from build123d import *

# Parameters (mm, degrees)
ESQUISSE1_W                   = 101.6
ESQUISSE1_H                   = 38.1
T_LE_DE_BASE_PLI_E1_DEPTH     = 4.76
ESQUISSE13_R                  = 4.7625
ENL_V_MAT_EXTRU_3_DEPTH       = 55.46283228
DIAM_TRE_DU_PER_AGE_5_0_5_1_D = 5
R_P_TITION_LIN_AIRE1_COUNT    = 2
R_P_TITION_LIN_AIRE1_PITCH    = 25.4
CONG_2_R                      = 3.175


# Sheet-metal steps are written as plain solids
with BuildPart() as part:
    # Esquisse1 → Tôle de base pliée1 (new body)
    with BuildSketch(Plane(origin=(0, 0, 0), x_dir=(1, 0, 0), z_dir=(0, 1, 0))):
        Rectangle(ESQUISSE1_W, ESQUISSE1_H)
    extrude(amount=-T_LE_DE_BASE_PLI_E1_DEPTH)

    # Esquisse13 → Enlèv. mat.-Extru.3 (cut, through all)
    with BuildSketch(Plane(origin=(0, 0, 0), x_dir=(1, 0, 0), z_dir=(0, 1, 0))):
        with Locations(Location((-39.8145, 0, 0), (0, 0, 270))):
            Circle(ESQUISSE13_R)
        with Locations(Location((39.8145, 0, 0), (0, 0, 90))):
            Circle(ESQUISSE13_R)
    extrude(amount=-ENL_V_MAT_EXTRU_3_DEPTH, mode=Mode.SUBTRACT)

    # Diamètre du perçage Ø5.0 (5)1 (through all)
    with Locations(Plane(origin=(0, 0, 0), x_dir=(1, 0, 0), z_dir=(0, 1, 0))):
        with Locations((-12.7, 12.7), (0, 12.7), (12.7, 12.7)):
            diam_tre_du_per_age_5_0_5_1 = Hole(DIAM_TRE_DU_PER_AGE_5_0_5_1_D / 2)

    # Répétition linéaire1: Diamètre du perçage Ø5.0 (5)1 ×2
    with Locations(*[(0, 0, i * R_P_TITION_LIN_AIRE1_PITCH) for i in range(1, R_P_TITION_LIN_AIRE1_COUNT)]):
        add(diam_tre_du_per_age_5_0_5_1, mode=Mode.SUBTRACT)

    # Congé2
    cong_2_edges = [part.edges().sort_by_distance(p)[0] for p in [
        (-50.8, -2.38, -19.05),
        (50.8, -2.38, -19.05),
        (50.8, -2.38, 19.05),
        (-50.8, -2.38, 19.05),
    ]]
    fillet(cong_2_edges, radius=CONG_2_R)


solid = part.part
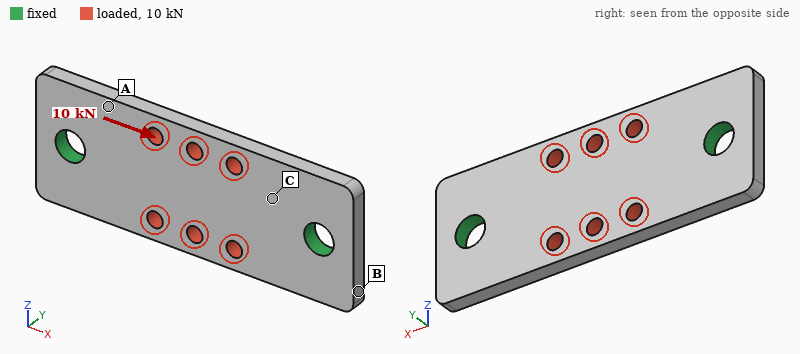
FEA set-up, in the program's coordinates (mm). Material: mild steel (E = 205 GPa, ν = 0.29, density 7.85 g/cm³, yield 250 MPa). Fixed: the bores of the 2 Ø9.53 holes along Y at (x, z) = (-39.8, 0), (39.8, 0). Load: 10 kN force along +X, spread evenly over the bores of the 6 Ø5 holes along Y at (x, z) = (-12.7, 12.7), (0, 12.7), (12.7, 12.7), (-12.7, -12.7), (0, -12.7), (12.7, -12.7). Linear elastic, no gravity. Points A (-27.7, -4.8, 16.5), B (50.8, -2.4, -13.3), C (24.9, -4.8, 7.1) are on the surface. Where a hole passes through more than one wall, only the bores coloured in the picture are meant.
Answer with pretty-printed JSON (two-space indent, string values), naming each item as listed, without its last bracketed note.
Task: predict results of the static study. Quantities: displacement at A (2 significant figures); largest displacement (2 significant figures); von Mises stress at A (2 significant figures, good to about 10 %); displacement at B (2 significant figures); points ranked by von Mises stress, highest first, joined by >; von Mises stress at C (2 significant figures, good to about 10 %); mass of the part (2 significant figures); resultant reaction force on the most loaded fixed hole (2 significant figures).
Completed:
{
  "displacement at A": "3.3 µm",
  "largest displacement": "6.3 µm",
  "von Mises stress at A": "19 MPa",
  "displacement at B": "2.2 µm",
  "points ranked by von Mises stress, highest first, joined by >": "C > A > B",
  "von Mises stress at C": "33 MPa",
  "mass of the part": "130 g",
  "resultant reaction force on the most loaded fixed hole": "5.0 kN"
}
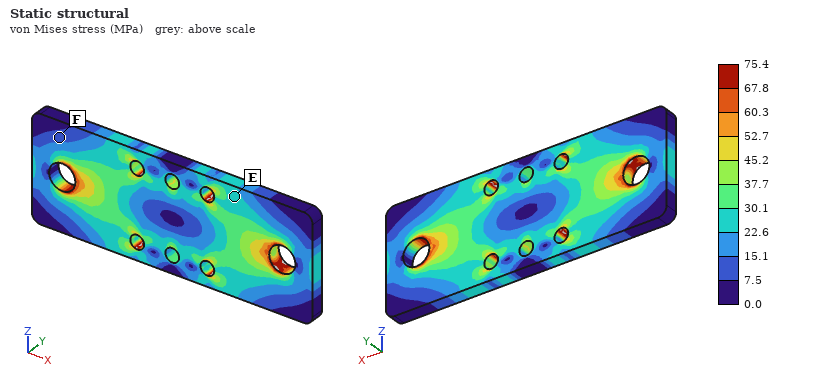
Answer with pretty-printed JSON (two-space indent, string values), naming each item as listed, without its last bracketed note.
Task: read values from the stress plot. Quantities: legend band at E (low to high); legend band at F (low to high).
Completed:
{
  "legend band at E": "22.6 to 30.1 MPa",
  "legend band at F": "7.5 to 15.1 MPa"
}
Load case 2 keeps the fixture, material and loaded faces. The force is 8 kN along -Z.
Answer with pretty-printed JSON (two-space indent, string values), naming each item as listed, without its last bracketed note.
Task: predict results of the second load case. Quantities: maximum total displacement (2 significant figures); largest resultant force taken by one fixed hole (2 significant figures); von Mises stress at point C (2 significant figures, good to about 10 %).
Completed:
{
  "maximum total displacement": "21 µm",
  "largest resultant force taken by one fixed hole": "4.0 kN",
  "von Mises stress at point C": "47 MPa"
}
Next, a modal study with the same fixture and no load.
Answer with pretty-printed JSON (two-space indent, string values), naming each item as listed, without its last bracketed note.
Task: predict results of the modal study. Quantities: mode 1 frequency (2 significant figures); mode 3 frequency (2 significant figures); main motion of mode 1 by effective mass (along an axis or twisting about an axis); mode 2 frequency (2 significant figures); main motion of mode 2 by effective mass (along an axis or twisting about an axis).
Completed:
{
  "mode 1 frequency": "4200 Hz",
  "mode 3 frequency": "10 kHz",
  "main motion of mode 1 by effective mass": "along Y",
  "mode 2 frequency": "5500 Hz",
  "main motion of mode 2 by effective mass": "twisting about X"
}
